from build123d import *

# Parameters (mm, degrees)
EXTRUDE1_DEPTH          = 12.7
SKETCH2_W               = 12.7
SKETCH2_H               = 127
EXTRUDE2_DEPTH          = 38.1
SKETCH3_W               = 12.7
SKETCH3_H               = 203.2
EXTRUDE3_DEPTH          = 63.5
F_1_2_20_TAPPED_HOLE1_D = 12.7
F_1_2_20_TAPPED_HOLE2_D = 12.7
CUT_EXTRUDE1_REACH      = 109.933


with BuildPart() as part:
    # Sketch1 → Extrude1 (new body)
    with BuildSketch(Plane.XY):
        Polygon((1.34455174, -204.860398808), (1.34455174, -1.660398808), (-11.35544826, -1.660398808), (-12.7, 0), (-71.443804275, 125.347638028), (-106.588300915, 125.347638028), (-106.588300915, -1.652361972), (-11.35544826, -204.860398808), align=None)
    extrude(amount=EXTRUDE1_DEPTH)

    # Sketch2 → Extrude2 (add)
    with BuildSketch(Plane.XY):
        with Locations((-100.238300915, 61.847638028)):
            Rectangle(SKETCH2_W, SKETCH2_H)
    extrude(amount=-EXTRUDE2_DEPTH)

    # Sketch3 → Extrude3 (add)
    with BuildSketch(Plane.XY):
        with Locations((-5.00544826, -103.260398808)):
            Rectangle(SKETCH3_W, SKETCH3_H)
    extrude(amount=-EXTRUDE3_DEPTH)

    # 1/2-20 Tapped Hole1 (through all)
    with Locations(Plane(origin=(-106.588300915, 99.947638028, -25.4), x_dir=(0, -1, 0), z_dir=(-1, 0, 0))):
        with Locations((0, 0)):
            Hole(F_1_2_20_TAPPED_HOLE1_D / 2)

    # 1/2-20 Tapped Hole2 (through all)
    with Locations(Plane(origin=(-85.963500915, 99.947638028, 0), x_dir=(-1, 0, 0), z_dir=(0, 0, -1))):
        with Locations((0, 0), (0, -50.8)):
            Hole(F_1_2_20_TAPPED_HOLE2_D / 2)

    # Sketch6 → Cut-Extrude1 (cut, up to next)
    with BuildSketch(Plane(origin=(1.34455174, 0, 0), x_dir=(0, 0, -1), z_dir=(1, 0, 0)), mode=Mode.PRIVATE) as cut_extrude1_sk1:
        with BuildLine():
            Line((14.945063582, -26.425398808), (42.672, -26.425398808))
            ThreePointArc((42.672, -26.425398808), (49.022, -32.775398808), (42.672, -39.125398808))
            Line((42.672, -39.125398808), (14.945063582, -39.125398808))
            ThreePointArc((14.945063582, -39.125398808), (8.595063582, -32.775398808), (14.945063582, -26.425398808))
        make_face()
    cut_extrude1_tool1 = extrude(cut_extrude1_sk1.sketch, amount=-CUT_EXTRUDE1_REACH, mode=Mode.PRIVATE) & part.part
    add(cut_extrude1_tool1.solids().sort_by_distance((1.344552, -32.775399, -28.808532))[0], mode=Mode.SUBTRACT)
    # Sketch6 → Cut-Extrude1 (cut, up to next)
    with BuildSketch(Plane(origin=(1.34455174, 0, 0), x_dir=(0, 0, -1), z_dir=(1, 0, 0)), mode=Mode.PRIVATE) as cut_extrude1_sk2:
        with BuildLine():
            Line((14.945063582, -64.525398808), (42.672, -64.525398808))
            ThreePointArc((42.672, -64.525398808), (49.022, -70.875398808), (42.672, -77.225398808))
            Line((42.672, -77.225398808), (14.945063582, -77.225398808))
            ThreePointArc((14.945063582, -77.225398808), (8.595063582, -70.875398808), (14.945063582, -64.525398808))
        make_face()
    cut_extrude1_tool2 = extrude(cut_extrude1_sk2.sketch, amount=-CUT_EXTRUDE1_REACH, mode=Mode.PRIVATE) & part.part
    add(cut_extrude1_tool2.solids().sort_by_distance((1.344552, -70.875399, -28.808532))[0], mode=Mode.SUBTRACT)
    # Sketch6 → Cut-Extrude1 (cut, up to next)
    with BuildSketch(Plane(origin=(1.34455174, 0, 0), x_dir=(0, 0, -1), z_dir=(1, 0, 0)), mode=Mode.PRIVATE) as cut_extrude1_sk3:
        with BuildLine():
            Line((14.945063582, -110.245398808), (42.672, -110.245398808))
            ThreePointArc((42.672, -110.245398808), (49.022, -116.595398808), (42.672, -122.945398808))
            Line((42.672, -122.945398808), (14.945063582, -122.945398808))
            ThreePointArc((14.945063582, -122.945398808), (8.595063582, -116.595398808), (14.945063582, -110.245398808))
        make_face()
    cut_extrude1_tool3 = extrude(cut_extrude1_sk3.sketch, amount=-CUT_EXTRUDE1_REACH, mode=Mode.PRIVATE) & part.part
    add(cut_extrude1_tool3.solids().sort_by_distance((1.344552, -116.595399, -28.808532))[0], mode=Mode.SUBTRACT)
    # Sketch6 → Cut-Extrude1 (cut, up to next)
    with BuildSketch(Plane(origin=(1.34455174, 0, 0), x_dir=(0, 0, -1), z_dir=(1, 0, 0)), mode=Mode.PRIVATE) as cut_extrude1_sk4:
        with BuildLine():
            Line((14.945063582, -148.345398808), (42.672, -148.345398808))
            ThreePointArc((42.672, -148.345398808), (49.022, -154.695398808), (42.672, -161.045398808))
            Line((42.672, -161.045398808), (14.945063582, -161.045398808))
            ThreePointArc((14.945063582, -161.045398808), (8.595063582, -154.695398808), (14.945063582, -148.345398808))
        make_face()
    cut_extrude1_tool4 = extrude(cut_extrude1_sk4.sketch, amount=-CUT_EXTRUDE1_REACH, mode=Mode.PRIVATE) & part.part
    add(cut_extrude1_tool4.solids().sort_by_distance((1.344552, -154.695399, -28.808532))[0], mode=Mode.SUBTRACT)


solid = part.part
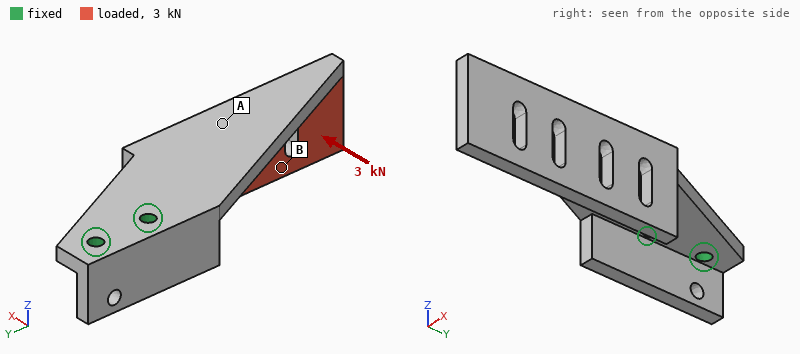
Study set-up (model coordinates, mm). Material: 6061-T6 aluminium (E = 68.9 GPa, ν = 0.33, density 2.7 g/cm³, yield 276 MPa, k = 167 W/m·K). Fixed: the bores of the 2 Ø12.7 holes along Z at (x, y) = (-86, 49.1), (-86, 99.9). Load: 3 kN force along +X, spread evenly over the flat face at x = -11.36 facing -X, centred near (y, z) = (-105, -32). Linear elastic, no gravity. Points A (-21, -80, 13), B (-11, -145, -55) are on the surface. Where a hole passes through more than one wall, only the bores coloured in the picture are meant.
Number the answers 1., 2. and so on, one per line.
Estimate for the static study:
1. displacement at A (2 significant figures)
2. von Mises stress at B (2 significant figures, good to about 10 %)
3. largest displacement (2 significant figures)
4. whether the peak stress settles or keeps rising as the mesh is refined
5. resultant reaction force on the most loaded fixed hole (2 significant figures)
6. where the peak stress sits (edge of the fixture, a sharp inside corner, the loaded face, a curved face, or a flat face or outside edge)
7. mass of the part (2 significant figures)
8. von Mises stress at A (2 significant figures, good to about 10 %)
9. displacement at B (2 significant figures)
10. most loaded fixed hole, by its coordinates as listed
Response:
1. 0.54 mm
2. 8.1 MPa
3. 1.9 mm
4. keeps rising
5. 10 kN
6. edge of the fixture
7. 1.2 kg
8. 28 MPa
9. 1.4 mm
10. (-86, 49.1)
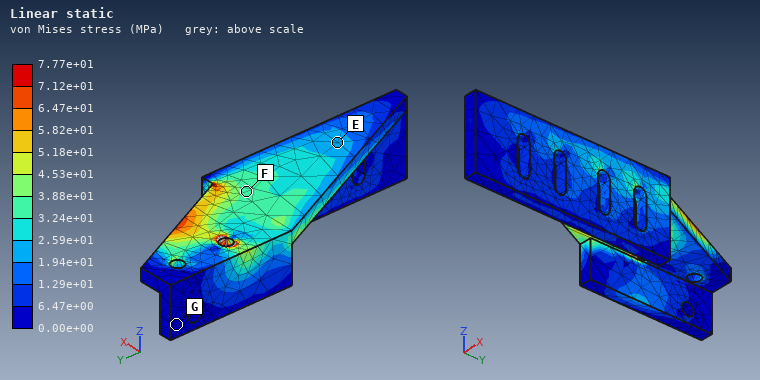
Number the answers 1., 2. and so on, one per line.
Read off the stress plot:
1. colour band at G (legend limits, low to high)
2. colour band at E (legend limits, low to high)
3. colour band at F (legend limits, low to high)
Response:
1. 0.00e+00 to 6.47e+00 MPa
2. 1.94e+01 to 2.59e+01 MPa
3. 3.24e+01 to 3.88e+01 MPa
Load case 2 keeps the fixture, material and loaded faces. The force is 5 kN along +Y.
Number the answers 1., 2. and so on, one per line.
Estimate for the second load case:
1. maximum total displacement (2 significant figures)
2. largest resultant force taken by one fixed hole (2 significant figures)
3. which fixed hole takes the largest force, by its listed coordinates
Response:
1. 3.6 mm
2. 8.0 kN
3. (-86, 99.9)
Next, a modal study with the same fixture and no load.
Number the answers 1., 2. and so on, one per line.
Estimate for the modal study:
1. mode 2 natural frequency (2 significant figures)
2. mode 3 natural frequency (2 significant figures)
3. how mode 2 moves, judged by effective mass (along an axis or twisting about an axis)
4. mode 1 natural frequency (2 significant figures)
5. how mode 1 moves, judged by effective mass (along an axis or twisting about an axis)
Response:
1. 460 Hz
2. 800 Hz
3. along X
4. 160 Hz
5. along Z
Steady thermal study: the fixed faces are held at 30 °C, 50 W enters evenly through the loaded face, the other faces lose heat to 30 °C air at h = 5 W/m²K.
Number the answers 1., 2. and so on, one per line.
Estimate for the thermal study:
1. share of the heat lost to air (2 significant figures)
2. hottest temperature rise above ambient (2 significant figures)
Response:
1. 17 %
2. 44 K
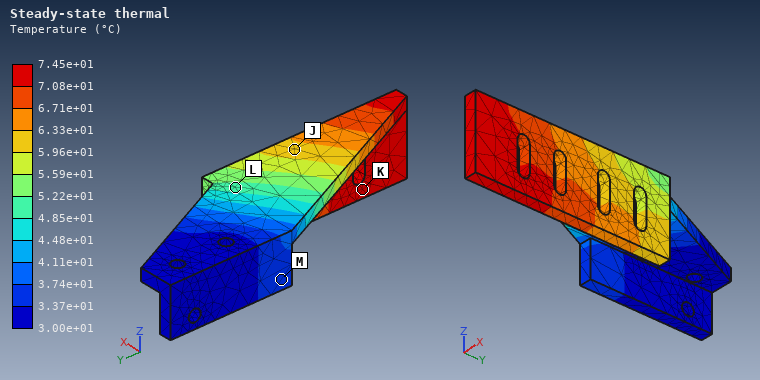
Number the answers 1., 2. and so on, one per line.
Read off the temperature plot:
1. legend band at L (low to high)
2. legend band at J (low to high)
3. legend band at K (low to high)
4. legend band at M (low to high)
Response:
1. 4.85e+01 to 5.22e+01 °C
2. 5.96e+01 to 6.33e+01 °C
3. 7.08e+01 to 7.45e+01 °C
4. 3.37e+01 to 3.74e+01 °C
